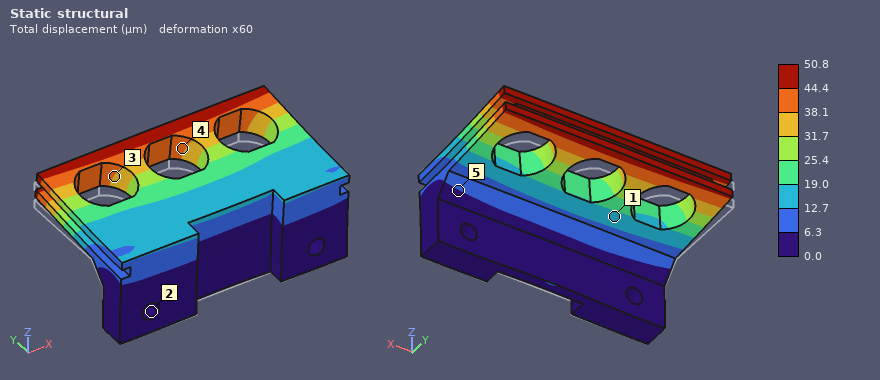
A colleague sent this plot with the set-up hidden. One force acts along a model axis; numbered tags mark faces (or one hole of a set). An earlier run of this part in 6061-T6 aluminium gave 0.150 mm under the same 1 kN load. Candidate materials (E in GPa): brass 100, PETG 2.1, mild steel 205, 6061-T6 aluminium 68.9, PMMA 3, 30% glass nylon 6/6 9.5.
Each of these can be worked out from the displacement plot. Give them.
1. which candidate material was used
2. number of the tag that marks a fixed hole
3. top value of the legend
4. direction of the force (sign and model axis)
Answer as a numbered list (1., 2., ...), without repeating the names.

1. mild steel
2. 2
3. 50.8 µm
4. +Z
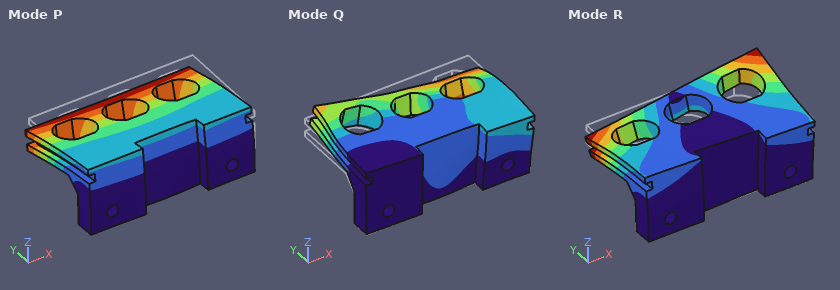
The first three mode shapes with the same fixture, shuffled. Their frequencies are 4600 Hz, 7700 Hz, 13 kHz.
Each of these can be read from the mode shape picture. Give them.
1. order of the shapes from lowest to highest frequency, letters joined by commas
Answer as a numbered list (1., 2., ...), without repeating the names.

1. P, R, Q
